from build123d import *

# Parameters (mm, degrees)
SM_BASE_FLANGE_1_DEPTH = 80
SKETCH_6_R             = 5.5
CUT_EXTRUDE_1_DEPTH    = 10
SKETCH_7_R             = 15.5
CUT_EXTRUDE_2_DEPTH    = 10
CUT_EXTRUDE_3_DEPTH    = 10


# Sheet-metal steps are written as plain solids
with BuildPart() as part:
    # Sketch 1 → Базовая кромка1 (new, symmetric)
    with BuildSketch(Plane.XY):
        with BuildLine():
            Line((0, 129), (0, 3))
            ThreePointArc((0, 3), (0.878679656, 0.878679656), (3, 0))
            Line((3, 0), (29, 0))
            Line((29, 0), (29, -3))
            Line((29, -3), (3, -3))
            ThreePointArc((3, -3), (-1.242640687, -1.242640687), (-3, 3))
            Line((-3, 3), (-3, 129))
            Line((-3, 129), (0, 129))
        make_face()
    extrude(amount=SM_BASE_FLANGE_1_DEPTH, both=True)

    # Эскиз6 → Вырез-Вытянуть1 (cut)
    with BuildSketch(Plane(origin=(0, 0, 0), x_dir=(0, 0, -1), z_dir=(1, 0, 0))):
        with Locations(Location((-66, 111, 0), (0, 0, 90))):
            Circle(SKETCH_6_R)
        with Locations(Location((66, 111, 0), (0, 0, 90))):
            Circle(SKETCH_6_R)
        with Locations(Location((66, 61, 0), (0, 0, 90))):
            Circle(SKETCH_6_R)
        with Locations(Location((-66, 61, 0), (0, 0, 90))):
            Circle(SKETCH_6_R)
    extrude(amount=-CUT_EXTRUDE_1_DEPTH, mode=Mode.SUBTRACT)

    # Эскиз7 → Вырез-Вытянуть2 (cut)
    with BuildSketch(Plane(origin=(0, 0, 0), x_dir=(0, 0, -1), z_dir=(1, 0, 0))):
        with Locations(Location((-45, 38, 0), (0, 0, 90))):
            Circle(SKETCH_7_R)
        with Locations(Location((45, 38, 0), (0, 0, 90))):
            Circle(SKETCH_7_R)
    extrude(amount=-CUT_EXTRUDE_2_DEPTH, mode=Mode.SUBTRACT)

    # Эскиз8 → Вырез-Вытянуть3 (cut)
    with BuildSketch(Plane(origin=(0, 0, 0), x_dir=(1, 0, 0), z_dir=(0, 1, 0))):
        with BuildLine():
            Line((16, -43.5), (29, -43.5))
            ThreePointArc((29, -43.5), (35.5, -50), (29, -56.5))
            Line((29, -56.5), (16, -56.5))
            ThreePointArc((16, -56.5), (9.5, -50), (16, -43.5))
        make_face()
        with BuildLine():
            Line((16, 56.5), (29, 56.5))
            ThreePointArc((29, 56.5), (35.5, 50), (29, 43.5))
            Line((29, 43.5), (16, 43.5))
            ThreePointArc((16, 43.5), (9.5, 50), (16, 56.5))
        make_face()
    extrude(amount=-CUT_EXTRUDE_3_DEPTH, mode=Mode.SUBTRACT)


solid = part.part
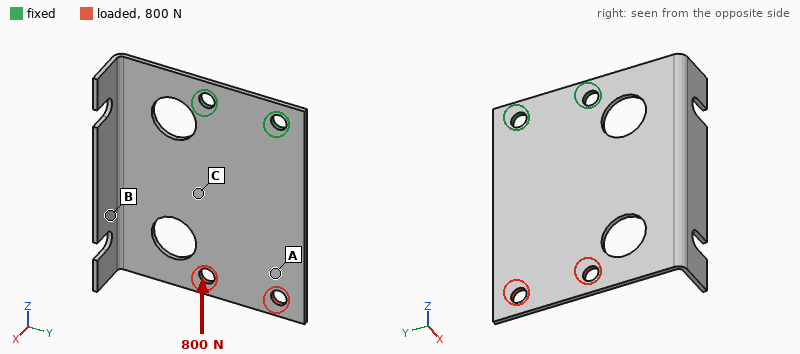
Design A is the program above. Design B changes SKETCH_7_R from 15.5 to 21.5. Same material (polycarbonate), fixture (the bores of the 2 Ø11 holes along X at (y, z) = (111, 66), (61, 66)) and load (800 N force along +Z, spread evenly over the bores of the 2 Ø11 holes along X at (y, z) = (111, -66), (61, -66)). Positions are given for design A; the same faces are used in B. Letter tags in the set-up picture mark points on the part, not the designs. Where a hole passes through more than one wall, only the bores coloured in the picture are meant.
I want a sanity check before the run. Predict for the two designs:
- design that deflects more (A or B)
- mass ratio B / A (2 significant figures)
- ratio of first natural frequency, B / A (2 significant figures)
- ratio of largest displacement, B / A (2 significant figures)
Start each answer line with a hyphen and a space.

- B
- 0.94
- 0.92
- 1.5
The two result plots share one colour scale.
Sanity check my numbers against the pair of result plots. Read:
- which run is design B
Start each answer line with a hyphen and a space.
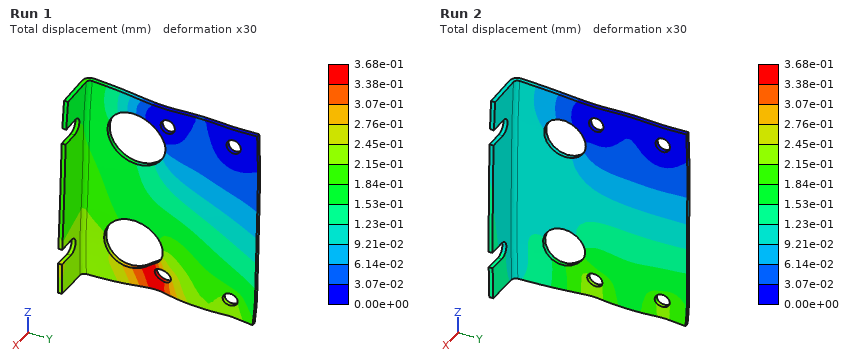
- Run 1
